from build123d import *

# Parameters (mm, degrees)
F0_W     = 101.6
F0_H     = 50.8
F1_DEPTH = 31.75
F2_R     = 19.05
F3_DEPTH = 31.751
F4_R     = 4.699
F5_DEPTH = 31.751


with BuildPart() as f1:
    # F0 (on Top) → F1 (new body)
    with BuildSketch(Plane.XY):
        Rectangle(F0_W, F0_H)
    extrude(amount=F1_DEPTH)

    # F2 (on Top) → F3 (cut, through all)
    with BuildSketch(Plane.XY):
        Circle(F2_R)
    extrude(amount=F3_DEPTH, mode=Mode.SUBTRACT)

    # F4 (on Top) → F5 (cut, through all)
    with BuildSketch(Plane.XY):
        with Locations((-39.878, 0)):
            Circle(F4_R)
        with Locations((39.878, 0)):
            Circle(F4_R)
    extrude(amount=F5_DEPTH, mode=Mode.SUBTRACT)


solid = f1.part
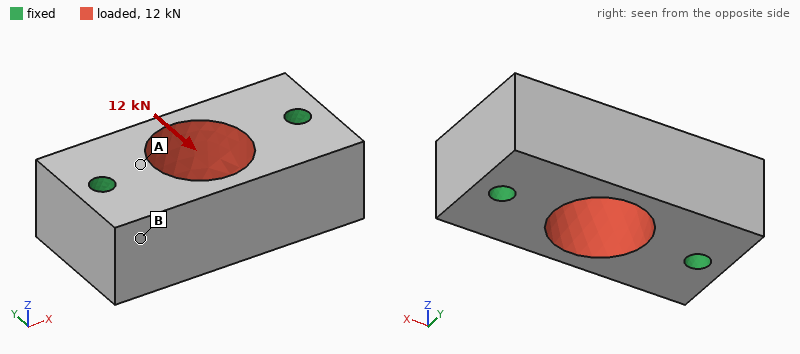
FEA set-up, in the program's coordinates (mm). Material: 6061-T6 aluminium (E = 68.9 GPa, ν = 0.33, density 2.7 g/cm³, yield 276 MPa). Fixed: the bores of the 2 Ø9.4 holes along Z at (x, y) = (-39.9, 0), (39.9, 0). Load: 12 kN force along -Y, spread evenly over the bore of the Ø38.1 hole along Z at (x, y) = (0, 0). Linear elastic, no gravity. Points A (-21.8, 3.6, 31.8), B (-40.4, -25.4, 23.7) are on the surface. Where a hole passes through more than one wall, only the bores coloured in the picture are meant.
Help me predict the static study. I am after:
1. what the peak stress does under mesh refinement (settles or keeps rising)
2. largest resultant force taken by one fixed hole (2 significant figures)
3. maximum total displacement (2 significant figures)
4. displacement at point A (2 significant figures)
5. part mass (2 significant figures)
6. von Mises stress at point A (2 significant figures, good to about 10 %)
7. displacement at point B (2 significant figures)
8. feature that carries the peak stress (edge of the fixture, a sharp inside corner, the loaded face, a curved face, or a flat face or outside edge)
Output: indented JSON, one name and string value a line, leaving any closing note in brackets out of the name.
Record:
{
  "what the peak stress does under mesh refinement": "keeps rising",
  "largest resultant force taken by one fixed hole": "6.0 kN",
  "maximum total displacement": "12 µm",
  "displacement at point A": "5.3 µm",
  "part mass": "330 g",
  "von Mises stress at point A": "9.7 MPa",
  "displacement at point B": "3.8 µm",
  "feature that carries the peak stress": "edge of the fixture"
}
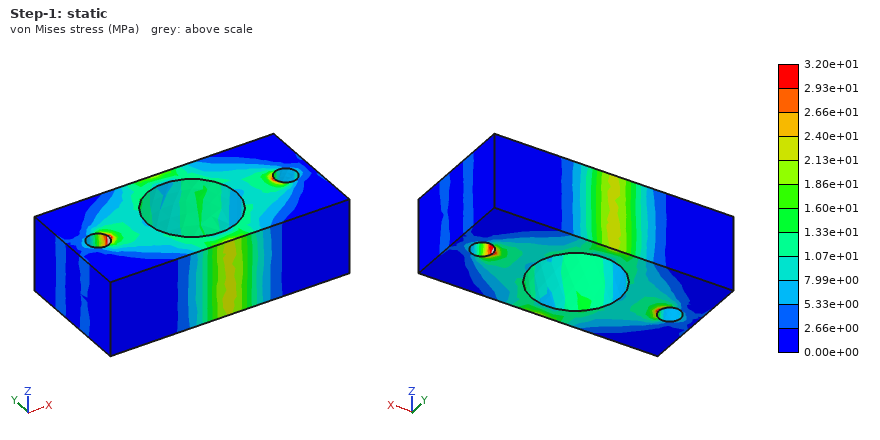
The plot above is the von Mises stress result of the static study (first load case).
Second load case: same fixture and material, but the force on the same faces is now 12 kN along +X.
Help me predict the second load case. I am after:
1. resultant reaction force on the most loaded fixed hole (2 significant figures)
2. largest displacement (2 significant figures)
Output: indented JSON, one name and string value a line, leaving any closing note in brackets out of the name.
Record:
{
  "resultant reaction force on the most loaded fixed hole": "6.0 kN",
  "largest displacement": "4.2 µm"
}
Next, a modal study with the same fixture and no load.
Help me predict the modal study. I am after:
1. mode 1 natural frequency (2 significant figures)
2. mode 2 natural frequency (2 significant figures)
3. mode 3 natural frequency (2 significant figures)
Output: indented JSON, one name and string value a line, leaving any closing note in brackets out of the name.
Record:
{
  "mode 1 natural frequency": "13 kHz",
  "mode 2 natural frequency": "15 kHz",
  "mode 3 natural frequency": "15 kHz"
}
